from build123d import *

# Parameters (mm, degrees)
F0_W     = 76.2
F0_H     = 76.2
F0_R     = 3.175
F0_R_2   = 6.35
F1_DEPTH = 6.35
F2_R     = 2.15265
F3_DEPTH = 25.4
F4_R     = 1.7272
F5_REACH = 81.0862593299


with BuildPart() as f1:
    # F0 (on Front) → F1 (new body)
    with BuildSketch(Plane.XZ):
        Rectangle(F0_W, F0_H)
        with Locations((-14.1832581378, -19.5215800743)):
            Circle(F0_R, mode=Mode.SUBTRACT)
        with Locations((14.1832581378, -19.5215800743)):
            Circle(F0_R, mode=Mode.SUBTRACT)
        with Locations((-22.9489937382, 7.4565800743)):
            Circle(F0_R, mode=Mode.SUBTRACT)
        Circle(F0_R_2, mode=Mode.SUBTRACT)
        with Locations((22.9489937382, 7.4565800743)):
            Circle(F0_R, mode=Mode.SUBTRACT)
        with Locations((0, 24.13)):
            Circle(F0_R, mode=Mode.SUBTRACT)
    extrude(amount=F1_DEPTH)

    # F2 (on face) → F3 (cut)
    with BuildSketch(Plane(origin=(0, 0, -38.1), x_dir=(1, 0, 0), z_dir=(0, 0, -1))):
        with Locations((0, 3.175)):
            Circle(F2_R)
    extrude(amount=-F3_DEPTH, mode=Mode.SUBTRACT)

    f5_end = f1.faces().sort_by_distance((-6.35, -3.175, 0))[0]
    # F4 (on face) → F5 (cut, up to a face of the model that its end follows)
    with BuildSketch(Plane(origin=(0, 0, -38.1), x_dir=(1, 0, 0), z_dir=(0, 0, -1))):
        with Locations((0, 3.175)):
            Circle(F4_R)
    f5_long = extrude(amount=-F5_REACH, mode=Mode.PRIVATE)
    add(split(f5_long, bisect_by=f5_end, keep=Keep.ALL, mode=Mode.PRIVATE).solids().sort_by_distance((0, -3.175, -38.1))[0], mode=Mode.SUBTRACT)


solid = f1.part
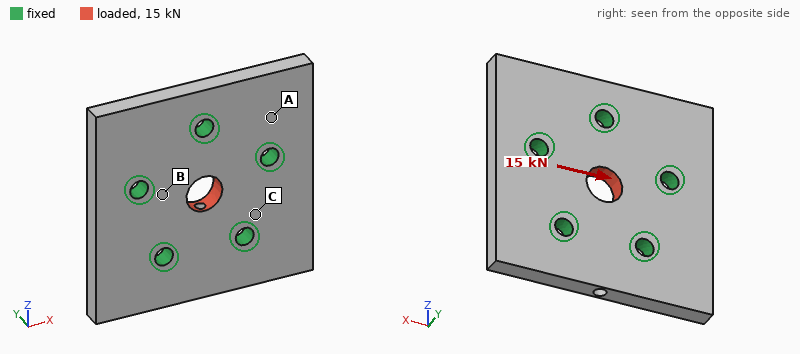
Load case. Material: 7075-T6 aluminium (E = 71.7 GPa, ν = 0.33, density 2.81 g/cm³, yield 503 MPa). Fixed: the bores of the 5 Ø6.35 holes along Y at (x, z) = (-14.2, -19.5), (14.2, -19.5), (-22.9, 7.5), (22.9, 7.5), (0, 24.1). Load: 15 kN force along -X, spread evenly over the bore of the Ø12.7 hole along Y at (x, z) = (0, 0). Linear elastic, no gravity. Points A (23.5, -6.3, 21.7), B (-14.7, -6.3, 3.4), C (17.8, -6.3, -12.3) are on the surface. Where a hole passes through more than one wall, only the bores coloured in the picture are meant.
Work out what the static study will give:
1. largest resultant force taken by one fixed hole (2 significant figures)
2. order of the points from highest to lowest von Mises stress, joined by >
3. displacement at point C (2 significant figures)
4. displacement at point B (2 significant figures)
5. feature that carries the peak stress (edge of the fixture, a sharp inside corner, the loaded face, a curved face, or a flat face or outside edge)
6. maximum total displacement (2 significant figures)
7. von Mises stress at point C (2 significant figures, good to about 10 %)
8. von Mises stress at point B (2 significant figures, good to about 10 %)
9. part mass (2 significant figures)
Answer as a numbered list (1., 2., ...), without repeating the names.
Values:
1. 4.4 kN
2. B > C > A
3. 3.5 µm
4. 5.4 µm
5. a curved face
6. 13 µm
7. 19 MPa
8. 57 MPa
9. 97 g
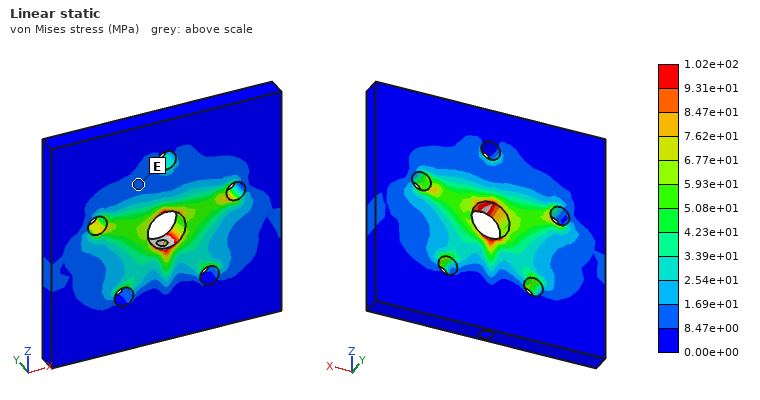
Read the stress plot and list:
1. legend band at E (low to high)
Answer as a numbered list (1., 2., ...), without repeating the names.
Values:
1. 8.47e+00 to 1.69e+01 MPa
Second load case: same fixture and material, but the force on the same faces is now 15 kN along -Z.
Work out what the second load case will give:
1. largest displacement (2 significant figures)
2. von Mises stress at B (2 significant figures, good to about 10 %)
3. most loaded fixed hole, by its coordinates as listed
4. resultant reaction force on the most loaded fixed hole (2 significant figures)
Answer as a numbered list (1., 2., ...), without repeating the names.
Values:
1. 13 µm
2. 21 MPa
3. (0, 24.1)
4. 4.6 kN
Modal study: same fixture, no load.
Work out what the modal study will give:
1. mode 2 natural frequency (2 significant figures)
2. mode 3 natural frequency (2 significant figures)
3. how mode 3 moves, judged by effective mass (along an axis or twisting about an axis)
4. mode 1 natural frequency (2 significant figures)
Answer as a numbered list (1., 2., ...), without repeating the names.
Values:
1. 8100 Hz
2. 9200 Hz
3. twisting about Z
4. 7800 Hz
